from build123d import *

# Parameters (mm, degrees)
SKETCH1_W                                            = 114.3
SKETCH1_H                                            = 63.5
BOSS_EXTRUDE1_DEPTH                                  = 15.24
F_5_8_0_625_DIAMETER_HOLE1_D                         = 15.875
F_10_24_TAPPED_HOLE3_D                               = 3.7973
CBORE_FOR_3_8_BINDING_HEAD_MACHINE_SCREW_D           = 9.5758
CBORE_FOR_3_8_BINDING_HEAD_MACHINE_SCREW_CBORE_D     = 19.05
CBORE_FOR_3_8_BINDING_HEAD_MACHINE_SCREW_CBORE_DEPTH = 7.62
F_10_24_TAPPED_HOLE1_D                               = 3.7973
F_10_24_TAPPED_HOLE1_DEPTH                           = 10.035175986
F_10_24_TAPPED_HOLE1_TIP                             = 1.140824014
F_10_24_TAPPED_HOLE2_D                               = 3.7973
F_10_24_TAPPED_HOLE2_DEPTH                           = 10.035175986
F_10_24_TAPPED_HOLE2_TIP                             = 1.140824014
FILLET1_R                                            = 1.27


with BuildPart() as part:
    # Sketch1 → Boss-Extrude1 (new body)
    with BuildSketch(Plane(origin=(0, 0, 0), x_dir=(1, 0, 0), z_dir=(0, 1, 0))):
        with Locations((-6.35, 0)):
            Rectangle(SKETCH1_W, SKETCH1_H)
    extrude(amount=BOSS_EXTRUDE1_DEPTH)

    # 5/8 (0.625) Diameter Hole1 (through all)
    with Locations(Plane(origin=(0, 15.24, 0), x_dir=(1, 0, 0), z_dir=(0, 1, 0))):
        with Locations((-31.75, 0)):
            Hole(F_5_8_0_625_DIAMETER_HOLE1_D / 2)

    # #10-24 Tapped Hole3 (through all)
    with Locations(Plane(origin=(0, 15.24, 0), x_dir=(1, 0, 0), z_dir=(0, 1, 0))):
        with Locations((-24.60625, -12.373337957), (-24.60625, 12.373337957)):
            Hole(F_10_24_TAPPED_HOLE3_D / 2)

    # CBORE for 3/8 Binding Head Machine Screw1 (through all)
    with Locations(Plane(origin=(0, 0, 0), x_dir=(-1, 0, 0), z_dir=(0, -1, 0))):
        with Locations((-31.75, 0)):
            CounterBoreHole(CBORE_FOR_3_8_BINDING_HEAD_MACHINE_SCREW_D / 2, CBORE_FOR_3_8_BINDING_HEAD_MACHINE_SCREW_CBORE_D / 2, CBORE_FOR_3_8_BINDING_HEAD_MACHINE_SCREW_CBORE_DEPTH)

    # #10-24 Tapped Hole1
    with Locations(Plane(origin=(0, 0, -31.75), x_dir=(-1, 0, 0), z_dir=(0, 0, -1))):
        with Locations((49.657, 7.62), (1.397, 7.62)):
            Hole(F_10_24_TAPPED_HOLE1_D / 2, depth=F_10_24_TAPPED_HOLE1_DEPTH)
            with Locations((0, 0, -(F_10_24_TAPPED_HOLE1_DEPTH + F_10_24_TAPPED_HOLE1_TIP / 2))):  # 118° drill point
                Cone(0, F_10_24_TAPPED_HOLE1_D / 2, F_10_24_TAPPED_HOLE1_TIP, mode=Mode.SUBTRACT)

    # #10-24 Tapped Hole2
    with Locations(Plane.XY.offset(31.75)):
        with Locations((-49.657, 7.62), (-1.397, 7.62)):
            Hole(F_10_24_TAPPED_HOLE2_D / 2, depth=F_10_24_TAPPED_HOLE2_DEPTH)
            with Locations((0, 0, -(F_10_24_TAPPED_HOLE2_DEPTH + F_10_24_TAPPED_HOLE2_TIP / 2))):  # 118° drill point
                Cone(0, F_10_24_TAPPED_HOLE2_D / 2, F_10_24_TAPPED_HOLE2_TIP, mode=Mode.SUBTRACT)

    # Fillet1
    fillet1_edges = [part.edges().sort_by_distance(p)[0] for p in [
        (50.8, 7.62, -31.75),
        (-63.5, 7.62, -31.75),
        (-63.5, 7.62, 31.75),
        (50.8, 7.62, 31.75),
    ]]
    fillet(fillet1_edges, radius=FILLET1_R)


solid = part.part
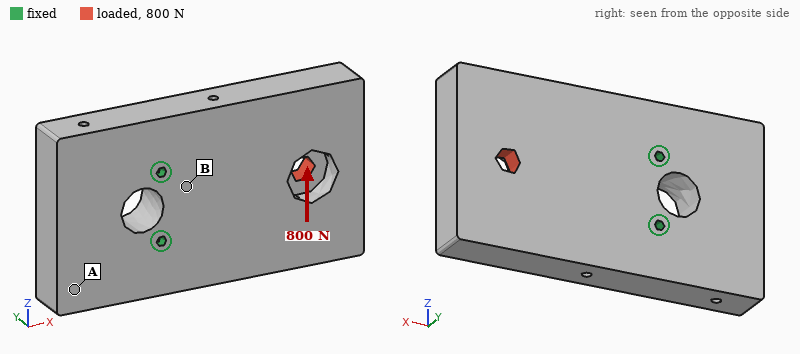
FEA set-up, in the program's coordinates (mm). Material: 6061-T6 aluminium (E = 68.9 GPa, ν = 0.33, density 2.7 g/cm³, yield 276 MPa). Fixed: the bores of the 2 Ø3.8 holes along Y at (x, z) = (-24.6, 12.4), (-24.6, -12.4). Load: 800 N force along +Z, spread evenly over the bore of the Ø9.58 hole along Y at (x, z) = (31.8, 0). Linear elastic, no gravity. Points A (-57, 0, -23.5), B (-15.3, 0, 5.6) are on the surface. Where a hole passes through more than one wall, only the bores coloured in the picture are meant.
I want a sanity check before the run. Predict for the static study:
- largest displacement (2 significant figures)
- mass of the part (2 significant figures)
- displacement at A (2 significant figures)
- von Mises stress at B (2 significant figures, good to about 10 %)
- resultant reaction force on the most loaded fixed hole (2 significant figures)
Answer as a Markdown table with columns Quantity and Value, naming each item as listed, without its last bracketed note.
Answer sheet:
| Quantity | Value |
|---|---|
| largest displacement | 13 µm |
| mass of the part | 280 g |
| displacement at A | 3.7 µm |
| von Mises stress at B | 4.0 MPa |
| resultant reaction force on the most loaded fixed hole | 1.7 kN |
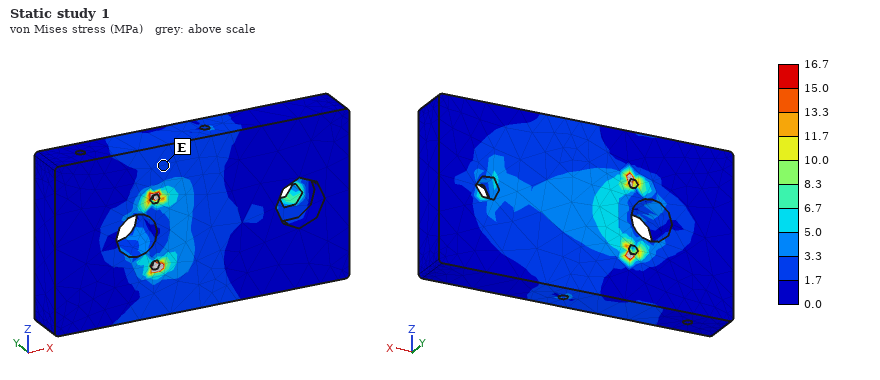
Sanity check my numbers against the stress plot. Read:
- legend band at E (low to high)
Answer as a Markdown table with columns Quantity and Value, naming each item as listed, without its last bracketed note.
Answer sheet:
| Quantity | Value |
|---|---|
| legend band at E | 1.7 to 3.3 MPa |
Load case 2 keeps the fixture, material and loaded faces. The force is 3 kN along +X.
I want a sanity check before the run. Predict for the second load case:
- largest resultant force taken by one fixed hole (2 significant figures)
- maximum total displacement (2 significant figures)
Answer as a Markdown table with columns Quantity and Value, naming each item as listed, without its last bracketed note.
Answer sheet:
| Quantity | Value |
|---|---|
| largest resultant force taken by one fixed hole | 1.5 kN |
| maximum total displacement | 29 µm |
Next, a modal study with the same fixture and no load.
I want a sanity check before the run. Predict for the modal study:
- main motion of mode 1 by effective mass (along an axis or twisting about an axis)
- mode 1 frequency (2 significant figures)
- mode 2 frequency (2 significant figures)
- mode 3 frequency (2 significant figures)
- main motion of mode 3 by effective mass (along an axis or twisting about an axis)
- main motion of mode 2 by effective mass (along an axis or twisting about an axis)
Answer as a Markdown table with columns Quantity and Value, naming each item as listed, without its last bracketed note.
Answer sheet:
| Quantity | Value |
|---|---|
| main motion of mode 1 by effective mass | along Y |
| mode 1 frequency | 1900 Hz |
| mode 2 frequency | 4100 Hz |
| mode 3 frequency | 4600 Hz |
| main motion of mode 3 by effective mass | twisting about X |
| main motion of mode 2 by effective mass | along Z |
